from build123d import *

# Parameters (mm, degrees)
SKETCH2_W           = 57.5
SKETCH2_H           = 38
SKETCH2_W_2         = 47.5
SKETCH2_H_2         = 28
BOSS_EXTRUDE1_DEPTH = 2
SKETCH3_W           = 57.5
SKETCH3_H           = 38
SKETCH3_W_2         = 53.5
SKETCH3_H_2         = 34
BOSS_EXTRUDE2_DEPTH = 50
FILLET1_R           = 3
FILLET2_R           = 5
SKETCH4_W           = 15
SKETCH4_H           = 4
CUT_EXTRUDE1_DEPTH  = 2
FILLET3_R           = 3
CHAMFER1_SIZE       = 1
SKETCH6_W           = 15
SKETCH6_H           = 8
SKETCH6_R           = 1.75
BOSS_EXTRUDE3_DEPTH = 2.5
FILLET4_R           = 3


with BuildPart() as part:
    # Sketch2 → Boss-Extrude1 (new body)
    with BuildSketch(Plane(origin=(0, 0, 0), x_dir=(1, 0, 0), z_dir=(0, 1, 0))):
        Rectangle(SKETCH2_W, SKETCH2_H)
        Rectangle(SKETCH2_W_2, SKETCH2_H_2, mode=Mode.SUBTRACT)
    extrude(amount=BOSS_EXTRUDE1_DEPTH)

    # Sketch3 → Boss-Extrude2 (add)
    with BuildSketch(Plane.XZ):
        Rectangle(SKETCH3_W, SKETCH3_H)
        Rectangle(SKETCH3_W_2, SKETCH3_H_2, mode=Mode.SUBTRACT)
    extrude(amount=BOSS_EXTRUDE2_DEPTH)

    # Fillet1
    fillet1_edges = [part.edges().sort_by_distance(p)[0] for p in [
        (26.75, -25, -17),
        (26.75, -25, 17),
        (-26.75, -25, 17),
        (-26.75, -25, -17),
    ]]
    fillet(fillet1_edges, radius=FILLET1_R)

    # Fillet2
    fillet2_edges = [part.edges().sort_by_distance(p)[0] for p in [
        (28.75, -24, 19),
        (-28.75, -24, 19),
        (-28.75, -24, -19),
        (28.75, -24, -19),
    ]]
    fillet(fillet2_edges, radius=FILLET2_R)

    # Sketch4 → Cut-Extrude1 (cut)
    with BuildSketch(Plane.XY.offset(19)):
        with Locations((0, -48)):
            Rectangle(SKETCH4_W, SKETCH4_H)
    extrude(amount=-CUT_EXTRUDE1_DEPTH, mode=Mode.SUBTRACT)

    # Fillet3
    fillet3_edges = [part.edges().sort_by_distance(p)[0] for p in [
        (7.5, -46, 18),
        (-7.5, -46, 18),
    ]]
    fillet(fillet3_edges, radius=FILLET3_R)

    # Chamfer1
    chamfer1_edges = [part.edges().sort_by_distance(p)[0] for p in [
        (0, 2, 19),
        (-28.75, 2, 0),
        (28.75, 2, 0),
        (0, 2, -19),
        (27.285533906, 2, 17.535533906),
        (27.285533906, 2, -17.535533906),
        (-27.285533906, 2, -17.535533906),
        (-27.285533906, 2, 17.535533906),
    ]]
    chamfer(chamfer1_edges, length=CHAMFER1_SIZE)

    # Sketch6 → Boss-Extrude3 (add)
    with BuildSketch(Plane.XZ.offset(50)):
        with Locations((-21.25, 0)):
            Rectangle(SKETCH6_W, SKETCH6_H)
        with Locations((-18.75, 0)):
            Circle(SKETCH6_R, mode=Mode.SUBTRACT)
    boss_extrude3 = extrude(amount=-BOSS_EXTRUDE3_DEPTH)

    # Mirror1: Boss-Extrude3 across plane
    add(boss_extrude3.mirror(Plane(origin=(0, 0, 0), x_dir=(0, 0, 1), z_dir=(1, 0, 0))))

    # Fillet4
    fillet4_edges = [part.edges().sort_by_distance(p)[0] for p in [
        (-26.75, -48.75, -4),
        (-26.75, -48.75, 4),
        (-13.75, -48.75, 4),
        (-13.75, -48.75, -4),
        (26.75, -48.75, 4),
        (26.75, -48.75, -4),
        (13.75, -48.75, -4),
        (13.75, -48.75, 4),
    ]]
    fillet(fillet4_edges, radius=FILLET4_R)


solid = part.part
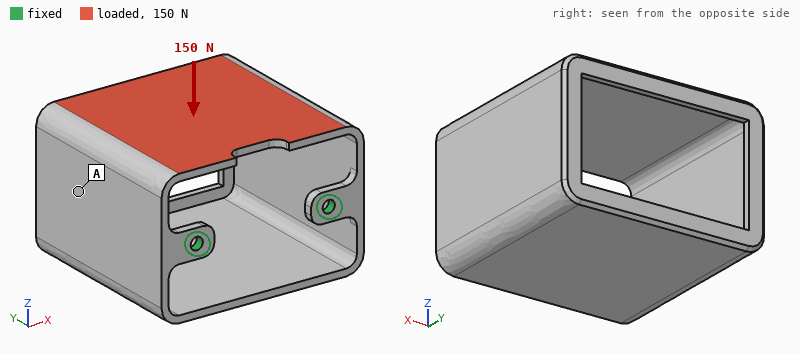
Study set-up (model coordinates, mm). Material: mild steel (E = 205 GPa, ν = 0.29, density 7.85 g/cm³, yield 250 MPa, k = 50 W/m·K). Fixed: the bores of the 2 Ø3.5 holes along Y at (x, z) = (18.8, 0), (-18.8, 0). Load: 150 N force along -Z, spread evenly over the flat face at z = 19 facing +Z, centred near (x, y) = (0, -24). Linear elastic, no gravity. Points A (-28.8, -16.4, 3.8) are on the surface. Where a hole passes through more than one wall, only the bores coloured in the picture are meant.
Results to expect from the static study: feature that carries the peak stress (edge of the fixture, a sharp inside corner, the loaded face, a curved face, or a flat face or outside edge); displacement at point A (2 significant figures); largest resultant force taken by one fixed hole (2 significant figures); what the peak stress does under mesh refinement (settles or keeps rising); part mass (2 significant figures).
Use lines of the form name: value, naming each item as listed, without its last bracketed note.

feature that carries the peak stress: edge of the fixture
displacement at point A: 0.13 mm
largest resultant force taken by one fixed hole: 78 N
what the peak stress does under mesh refinement: keeps rising
part mass: 150 g
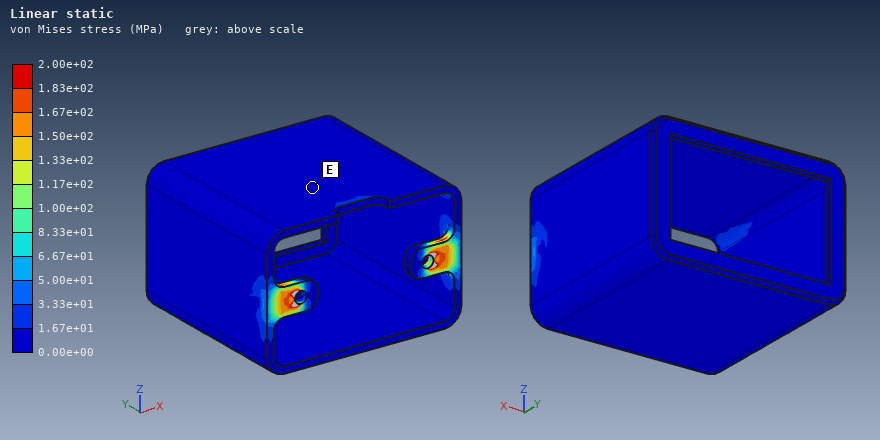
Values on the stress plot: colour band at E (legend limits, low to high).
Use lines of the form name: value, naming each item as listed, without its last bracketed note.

colour band at E: 0.00e+00 to 1.67e+01 MPa
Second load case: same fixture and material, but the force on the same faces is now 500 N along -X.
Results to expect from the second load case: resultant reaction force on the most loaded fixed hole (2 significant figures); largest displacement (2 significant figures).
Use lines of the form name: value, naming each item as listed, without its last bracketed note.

resultant reaction force on the most loaded fixed hole: 350 N
largest displacement: 0.11 mm
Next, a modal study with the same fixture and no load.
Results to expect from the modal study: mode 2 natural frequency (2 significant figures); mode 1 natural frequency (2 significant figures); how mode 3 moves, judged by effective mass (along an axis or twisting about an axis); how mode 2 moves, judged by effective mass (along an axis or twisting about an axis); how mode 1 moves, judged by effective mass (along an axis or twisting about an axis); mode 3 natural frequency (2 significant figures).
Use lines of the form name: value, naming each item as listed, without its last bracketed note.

mode 2 natural frequency: 1100 Hz
mode 1 natural frequency: 370 Hz
how mode 3 moves, judged by effective mass: twisting about Y
how mode 2 moves, judged by effective mass: along X
how mode 1 moves, judged by effective mass: along Z
mode 3 natural frequency: 1600 Hz
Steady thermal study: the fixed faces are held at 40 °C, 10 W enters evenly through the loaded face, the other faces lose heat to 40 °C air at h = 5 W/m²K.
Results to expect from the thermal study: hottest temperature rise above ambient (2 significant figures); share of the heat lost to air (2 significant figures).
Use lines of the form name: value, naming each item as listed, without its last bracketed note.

hottest temperature rise above ambient: 64 K
share of the heat lost to air: 37 %
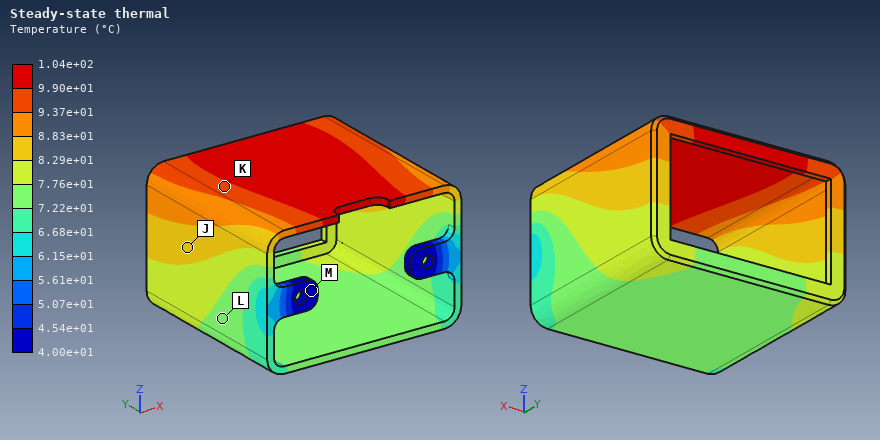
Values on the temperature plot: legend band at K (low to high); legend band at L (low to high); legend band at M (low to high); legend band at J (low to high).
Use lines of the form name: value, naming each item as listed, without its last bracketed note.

legend band at K: 9.37e+01 to 9.90e+01 °C
legend band at L: 7.22e+01 to 7.76e+01 °C
legend band at M: 4.00e+01 to 4.54e+01 °C
legend band at J: 8.29e+01 to 8.83e+01 °C
